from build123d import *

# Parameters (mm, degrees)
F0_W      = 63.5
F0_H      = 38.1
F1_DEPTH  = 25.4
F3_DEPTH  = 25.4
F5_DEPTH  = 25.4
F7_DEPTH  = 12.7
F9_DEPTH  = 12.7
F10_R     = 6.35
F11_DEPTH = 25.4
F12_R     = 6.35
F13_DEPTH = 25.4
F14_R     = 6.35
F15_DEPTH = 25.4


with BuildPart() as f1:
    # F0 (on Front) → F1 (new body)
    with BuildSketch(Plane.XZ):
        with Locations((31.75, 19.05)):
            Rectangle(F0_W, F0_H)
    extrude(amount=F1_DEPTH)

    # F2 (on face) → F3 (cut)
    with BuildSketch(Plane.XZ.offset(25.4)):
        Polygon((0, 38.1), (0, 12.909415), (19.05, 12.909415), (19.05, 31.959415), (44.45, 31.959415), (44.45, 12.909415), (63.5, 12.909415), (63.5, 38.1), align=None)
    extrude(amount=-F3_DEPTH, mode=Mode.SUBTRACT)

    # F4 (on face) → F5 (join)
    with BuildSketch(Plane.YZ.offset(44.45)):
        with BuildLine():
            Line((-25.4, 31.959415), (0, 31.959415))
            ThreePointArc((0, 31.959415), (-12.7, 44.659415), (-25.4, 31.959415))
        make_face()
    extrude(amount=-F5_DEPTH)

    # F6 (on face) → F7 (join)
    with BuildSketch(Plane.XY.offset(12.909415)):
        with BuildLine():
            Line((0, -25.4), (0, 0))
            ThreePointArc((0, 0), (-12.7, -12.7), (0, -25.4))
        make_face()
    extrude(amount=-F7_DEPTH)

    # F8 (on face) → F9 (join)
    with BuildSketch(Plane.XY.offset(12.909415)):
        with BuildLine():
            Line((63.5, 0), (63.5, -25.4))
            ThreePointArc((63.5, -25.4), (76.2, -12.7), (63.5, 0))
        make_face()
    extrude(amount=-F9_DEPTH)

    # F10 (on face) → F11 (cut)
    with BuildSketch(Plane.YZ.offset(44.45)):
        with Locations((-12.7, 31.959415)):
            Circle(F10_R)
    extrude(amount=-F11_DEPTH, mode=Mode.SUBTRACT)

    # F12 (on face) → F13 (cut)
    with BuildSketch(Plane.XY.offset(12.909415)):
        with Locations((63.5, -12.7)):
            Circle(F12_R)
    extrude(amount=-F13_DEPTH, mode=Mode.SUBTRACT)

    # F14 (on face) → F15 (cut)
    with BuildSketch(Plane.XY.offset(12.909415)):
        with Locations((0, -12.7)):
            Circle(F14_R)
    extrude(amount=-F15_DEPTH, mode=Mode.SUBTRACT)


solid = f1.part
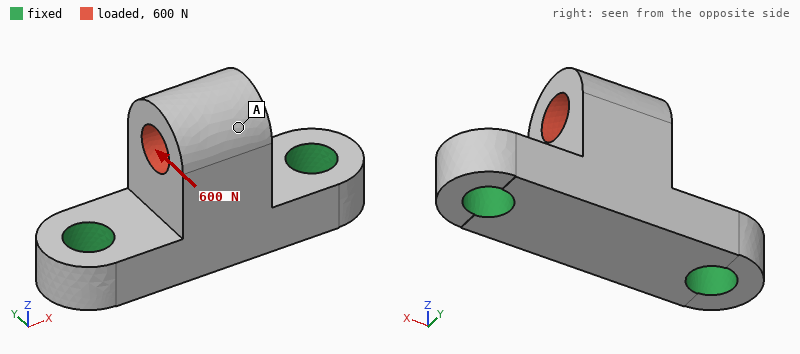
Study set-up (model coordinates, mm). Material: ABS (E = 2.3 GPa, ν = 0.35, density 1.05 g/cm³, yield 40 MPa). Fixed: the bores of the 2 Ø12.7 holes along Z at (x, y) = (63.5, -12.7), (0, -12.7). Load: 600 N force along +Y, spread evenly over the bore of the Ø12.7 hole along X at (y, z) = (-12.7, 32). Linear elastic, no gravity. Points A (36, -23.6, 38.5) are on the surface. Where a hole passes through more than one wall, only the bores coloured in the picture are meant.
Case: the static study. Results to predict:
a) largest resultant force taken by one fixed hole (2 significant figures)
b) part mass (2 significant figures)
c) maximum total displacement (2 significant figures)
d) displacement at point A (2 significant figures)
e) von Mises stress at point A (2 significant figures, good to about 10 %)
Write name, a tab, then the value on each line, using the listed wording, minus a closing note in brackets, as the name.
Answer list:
largest resultant force taken by one fixed hole	300 N
part mass	41 g
maximum total displacement	0.57 mm
displacement at point A	0.51 mm
von Mises stress at point A	1.6 MPa
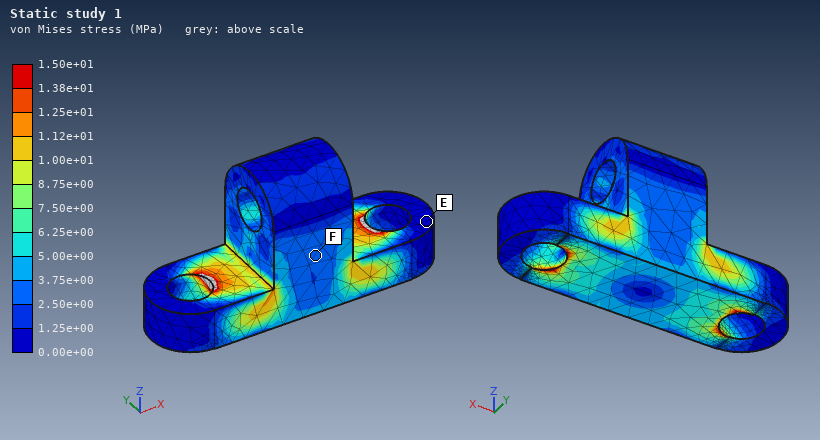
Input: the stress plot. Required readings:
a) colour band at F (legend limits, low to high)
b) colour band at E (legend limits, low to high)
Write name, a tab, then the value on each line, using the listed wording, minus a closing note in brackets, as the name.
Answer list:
colour band at F	2.50e+00 to 3.75e+00 MPa
colour band at E	0.00e+00 to 1.25e+00 MPa
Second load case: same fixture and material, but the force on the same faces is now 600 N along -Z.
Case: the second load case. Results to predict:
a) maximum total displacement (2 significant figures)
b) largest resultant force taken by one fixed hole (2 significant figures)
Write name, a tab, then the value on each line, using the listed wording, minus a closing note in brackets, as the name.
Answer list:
maximum total displacement	62 µm
largest resultant force taken by one fixed hole	310 N
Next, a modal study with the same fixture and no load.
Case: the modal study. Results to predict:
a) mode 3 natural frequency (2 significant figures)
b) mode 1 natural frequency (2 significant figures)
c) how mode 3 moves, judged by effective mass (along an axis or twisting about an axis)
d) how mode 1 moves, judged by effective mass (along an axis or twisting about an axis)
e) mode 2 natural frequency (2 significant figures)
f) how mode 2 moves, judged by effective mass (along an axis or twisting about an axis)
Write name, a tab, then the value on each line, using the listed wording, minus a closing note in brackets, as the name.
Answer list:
mode 3 natural frequency	3500 Hz
mode 1 natural frequency	1700 Hz
how mode 3 moves, judged by effective mass	along Z
how mode 1 moves, judged by effective mass	along Y
mode 2 natural frequency	3100 Hz
how mode 2 moves, judged by effective mass	along X
